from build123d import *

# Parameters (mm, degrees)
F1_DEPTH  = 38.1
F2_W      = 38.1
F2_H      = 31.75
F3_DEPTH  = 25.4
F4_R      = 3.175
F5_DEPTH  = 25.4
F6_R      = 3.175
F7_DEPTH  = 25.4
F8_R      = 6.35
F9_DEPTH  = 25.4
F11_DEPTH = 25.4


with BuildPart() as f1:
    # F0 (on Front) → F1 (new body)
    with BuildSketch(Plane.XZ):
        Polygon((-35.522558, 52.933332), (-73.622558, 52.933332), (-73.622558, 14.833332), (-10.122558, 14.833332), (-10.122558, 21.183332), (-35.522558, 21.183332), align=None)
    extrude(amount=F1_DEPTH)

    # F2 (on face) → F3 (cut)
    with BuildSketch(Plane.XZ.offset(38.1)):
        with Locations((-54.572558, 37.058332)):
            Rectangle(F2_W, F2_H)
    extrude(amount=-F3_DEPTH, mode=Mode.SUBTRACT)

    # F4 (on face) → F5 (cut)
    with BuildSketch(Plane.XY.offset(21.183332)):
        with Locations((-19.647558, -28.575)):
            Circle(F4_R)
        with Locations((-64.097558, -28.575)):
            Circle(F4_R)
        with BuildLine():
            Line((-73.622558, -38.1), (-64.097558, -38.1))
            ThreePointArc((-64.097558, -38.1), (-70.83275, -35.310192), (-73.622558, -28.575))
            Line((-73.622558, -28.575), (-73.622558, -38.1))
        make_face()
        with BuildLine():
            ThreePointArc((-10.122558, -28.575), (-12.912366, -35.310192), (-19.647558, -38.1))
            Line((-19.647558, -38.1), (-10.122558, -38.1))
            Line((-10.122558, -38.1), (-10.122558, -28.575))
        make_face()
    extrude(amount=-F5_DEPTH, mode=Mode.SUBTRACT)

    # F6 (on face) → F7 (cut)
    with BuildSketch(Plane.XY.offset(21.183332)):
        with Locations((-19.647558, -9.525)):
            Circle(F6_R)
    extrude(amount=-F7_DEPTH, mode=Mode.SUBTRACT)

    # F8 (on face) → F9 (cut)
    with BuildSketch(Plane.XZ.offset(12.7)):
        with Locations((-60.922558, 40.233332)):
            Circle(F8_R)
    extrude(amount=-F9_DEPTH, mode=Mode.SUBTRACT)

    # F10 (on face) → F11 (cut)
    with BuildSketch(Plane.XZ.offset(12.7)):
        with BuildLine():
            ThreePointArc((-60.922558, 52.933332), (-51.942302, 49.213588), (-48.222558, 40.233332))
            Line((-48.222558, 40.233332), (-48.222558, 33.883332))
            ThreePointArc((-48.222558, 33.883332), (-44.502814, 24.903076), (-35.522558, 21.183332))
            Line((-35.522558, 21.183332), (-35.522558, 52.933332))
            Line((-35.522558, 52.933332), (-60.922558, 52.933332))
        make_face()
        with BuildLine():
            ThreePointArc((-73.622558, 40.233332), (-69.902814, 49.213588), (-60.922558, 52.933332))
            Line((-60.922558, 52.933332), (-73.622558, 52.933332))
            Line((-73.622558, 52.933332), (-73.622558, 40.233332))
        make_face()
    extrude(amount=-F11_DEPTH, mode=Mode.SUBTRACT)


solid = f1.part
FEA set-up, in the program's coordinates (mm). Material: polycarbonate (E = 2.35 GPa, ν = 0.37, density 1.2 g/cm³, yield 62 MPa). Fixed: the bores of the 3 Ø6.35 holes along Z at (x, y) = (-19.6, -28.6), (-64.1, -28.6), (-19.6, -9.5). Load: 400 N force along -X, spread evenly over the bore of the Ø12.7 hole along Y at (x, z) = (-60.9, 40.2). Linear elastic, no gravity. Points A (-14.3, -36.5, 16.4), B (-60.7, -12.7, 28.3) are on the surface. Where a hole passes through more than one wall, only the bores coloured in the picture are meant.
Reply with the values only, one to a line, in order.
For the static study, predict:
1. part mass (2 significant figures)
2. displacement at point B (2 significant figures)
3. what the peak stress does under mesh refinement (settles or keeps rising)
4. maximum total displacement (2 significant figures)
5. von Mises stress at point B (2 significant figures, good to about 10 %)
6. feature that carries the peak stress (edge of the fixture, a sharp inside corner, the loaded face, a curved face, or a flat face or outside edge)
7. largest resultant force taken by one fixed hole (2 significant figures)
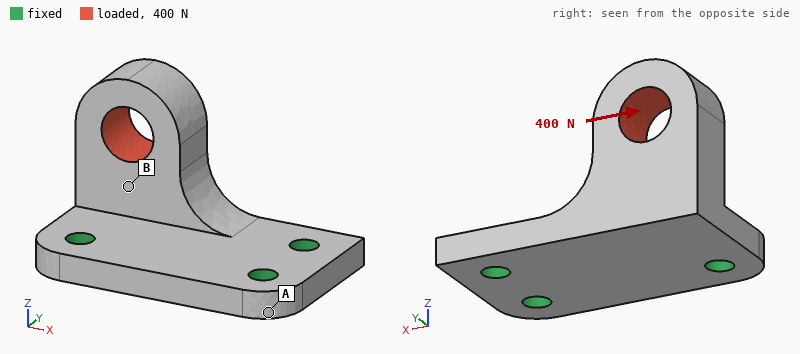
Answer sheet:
27 g
0.28 mm
keeps rising
0.87 mm
6.5 MPa
edge of the fixture
260 N
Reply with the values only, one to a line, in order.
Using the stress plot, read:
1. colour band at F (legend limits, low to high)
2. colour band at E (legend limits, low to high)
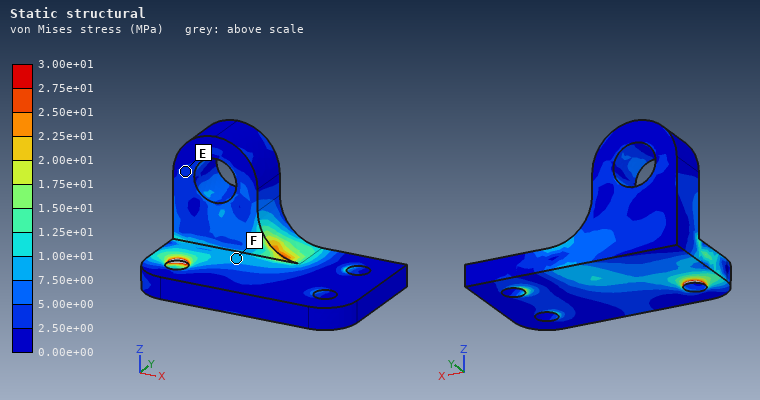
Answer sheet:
7.50e+00 to 1.00e+01 MPa
2.50e+00 to 5.00e+00 MPa
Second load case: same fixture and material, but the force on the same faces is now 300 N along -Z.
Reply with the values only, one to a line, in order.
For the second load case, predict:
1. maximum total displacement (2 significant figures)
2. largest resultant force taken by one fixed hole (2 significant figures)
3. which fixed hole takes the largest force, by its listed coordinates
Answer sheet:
0.97 mm
240 N
(-64.1, -28.6)
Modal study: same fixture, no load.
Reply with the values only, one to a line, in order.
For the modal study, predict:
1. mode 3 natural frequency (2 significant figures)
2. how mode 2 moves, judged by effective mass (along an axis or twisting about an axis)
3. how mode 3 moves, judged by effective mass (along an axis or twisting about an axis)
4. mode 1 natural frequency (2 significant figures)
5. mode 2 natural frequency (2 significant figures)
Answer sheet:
2500 Hz
along X
along Z
820 Hz
1800 Hz
